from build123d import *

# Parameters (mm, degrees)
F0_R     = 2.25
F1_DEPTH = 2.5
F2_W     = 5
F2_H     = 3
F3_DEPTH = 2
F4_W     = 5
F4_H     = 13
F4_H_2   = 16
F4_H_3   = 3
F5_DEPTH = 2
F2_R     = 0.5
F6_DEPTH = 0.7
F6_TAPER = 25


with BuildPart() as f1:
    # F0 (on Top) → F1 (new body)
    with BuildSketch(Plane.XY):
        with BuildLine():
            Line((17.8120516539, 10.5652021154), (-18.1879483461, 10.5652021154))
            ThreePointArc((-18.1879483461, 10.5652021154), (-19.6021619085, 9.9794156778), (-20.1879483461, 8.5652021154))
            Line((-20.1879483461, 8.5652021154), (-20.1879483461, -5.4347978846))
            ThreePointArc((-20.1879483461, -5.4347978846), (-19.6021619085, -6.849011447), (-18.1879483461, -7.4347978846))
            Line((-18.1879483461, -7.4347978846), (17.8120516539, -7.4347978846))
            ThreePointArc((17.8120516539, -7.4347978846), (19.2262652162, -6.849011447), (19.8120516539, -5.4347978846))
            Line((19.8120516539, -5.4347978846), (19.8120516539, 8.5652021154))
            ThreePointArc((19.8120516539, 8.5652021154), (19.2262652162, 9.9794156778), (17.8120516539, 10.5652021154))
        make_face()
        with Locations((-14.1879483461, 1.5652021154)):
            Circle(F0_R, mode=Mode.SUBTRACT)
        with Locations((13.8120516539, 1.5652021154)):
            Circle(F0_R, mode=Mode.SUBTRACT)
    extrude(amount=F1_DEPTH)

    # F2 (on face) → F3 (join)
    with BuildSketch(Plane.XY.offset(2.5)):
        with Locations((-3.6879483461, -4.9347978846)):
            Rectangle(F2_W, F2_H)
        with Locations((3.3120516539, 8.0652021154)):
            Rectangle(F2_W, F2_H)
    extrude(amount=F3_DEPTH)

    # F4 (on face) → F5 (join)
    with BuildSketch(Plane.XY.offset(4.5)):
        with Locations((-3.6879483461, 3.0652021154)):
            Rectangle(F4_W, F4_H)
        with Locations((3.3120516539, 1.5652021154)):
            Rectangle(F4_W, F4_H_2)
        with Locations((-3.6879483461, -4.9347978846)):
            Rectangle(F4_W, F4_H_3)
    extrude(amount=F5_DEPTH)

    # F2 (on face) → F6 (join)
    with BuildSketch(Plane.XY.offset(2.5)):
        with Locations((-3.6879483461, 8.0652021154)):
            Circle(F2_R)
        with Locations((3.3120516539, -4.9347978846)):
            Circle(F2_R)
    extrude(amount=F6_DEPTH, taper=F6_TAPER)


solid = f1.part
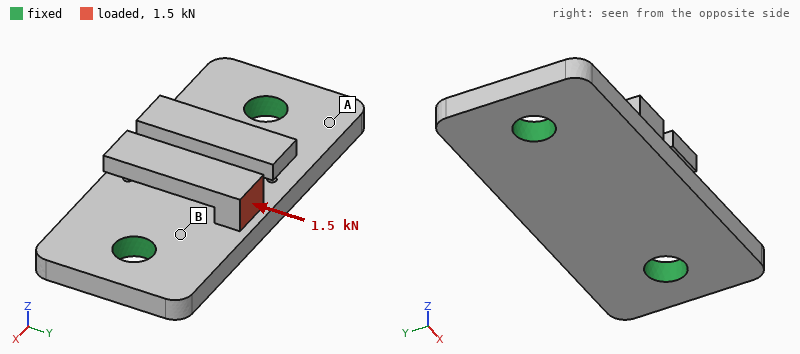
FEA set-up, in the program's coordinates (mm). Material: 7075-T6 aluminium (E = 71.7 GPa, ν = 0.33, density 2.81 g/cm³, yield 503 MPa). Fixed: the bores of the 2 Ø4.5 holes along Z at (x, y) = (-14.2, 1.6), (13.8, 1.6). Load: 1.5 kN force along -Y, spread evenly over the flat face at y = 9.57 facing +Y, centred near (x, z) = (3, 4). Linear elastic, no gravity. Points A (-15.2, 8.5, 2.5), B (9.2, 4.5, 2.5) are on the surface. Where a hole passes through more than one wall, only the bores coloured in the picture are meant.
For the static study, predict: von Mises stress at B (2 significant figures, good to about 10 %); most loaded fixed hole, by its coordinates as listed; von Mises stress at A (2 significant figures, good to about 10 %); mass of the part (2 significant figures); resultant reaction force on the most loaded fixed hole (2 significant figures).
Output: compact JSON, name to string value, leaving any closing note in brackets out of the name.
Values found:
{"von Mises stress at B": "220 MPa", "most loaded fixed hole, by its coordinates as listed": "(13.8, 1.6)", "von Mises stress at A": "49 MPa", "mass of the part": "5.9 g", "resultant reaction force on the most loaded fixed hole": "970 N"}
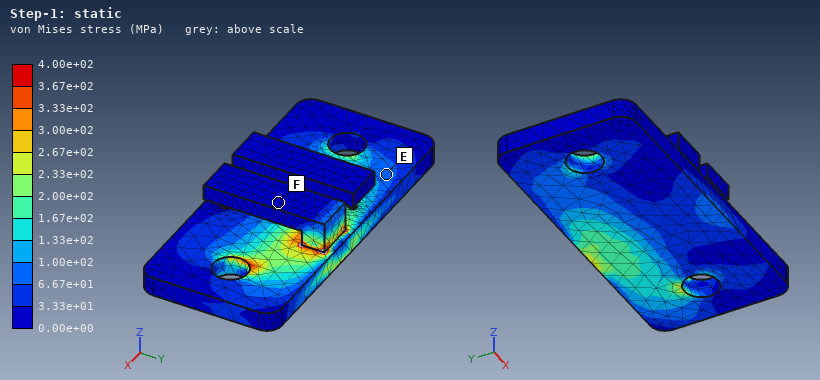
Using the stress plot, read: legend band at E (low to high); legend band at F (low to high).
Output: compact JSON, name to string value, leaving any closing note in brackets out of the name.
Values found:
{"legend band at E": "6.67e+01 to 1.00e+02 MPa", "legend band at F": "0.00e+00 to 3.33e+01 MPa"}
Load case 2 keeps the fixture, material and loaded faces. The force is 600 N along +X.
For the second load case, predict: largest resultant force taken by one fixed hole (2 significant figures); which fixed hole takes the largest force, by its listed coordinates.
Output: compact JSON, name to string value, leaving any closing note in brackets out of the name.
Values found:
{"largest resultant force taken by one fixed hole": "400 N", "which fixed hole takes the largest force, by its listed coordinates": "(13.8, 1.6)"}
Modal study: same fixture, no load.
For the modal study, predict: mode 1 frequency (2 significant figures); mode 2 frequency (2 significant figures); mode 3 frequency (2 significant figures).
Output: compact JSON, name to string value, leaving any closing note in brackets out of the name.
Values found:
{"mode 1 frequency": "6800 Hz", "mode 2 frequency": "6900 Hz", "mode 3 frequency": "11 kHz"}
